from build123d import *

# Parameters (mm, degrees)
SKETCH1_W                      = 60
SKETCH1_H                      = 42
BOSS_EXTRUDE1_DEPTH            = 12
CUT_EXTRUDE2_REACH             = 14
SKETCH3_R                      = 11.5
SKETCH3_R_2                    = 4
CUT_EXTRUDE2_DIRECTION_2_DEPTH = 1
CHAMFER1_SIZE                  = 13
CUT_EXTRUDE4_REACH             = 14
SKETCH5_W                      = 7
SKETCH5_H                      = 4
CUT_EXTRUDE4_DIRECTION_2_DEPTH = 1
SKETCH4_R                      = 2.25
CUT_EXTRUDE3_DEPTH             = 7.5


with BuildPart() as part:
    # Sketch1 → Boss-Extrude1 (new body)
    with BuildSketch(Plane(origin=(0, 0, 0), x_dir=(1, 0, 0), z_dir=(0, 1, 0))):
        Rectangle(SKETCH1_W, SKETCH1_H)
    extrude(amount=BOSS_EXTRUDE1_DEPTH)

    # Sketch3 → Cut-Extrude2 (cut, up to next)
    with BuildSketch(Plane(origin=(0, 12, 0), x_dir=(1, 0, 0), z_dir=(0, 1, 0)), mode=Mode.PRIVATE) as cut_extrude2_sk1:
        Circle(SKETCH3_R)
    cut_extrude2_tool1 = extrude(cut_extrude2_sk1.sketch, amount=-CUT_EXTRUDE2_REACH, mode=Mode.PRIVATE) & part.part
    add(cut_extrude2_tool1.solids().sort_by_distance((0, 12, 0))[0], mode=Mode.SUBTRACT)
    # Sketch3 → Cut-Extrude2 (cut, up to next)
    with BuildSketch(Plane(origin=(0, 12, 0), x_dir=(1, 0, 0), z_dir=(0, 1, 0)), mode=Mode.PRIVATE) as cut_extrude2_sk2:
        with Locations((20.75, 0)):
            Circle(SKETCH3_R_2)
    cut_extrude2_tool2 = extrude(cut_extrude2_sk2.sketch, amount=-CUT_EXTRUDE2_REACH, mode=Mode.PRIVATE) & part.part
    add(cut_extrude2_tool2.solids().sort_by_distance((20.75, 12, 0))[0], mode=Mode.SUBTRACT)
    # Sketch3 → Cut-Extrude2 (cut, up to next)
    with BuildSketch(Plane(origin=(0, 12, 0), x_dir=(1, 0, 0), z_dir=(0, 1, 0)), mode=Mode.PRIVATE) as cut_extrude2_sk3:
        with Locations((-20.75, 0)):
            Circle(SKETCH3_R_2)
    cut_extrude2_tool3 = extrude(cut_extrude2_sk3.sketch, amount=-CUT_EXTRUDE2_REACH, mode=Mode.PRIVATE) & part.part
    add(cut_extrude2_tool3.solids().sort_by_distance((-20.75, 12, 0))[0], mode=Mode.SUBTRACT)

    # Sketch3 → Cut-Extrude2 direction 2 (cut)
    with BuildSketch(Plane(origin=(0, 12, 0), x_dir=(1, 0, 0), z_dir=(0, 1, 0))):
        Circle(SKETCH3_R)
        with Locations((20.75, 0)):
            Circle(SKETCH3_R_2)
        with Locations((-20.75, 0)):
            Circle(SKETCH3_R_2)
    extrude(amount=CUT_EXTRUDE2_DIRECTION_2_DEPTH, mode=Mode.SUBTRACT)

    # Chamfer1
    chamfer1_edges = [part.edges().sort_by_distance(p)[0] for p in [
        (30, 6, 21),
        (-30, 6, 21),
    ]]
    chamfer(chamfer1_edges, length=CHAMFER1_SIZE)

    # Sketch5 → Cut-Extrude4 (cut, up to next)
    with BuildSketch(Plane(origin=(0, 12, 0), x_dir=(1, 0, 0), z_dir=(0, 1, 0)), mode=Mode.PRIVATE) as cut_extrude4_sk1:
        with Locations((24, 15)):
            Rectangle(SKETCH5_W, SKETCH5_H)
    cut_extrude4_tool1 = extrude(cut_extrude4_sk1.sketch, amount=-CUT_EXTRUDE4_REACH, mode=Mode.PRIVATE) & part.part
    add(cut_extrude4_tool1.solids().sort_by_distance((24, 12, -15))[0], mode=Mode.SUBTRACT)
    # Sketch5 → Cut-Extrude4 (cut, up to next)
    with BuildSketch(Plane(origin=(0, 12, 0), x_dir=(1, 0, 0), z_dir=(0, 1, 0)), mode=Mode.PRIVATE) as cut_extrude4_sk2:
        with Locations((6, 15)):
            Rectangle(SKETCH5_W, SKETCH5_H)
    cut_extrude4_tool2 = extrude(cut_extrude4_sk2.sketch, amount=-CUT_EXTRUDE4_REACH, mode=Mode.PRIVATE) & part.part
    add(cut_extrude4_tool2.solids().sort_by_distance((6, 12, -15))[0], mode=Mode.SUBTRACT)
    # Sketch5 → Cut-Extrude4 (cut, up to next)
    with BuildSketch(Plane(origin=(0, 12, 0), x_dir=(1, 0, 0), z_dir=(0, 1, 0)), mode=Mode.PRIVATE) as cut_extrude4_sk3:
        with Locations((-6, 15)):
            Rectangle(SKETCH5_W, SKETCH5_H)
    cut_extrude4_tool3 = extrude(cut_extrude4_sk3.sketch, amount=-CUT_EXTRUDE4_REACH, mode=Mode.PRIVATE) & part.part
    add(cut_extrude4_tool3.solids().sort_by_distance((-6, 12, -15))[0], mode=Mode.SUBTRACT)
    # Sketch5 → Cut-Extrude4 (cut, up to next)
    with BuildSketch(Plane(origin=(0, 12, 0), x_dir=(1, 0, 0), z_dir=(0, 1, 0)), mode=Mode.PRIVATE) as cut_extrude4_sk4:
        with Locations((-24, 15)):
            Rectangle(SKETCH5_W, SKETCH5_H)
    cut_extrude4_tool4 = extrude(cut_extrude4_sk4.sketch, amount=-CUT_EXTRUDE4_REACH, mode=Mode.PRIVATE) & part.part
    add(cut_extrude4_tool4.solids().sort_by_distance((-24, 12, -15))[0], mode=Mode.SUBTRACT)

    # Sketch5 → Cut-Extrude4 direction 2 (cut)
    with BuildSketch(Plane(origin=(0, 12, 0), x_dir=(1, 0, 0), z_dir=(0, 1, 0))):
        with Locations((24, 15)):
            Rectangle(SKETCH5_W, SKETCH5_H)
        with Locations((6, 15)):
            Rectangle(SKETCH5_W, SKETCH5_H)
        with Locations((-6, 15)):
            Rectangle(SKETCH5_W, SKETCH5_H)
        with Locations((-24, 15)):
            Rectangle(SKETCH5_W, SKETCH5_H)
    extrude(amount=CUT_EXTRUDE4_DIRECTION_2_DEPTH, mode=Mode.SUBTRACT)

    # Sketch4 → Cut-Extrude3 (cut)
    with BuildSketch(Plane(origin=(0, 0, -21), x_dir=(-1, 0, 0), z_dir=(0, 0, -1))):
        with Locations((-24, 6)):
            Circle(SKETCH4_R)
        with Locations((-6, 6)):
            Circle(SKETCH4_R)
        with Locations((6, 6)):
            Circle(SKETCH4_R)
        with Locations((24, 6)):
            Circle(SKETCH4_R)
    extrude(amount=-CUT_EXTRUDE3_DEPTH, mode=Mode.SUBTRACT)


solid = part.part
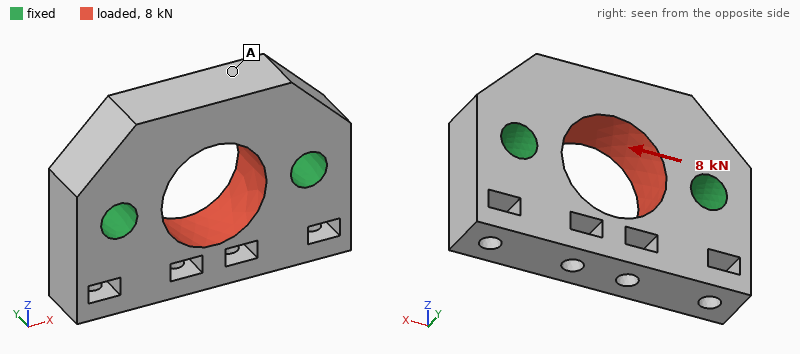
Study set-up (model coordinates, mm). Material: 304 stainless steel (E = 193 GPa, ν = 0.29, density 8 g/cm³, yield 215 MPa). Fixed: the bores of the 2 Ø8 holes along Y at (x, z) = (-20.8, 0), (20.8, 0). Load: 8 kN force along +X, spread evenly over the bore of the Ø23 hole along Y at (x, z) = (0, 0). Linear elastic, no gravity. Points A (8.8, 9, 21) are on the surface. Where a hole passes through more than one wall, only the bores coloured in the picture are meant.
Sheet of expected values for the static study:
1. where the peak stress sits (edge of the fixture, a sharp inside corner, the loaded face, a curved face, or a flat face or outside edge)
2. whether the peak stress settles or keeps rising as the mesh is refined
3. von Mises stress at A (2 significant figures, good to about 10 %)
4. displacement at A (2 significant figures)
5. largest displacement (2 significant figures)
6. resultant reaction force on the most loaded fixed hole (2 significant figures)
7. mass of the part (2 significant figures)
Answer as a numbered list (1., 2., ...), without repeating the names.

1. edge of the fixture
2. keeps rising
3. 6.4 MPa
4. 1.4 µm
5. 2.3 µm
6. 4.0 kN
7. 160 g
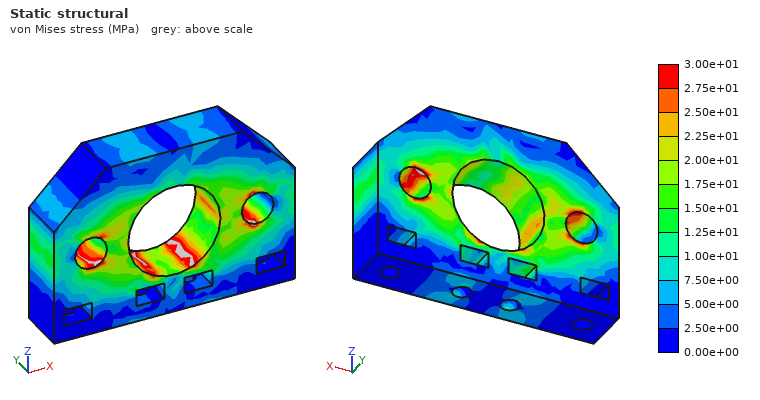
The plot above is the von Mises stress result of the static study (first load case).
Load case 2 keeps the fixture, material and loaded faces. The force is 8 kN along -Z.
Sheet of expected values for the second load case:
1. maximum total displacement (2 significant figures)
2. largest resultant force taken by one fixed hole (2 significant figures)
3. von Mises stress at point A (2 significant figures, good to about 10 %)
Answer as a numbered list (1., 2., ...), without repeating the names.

1. 5.0 µm
2. 4.0 kN
3. 11 MPa
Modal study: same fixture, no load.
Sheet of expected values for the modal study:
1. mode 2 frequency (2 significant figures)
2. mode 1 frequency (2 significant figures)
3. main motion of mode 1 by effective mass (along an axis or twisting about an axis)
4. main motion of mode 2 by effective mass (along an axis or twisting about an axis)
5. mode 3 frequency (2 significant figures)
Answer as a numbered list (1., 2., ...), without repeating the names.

1. 17 kHz
2. 16 kHz
3. twisting about X
4. along Y
5. 22 kHz
